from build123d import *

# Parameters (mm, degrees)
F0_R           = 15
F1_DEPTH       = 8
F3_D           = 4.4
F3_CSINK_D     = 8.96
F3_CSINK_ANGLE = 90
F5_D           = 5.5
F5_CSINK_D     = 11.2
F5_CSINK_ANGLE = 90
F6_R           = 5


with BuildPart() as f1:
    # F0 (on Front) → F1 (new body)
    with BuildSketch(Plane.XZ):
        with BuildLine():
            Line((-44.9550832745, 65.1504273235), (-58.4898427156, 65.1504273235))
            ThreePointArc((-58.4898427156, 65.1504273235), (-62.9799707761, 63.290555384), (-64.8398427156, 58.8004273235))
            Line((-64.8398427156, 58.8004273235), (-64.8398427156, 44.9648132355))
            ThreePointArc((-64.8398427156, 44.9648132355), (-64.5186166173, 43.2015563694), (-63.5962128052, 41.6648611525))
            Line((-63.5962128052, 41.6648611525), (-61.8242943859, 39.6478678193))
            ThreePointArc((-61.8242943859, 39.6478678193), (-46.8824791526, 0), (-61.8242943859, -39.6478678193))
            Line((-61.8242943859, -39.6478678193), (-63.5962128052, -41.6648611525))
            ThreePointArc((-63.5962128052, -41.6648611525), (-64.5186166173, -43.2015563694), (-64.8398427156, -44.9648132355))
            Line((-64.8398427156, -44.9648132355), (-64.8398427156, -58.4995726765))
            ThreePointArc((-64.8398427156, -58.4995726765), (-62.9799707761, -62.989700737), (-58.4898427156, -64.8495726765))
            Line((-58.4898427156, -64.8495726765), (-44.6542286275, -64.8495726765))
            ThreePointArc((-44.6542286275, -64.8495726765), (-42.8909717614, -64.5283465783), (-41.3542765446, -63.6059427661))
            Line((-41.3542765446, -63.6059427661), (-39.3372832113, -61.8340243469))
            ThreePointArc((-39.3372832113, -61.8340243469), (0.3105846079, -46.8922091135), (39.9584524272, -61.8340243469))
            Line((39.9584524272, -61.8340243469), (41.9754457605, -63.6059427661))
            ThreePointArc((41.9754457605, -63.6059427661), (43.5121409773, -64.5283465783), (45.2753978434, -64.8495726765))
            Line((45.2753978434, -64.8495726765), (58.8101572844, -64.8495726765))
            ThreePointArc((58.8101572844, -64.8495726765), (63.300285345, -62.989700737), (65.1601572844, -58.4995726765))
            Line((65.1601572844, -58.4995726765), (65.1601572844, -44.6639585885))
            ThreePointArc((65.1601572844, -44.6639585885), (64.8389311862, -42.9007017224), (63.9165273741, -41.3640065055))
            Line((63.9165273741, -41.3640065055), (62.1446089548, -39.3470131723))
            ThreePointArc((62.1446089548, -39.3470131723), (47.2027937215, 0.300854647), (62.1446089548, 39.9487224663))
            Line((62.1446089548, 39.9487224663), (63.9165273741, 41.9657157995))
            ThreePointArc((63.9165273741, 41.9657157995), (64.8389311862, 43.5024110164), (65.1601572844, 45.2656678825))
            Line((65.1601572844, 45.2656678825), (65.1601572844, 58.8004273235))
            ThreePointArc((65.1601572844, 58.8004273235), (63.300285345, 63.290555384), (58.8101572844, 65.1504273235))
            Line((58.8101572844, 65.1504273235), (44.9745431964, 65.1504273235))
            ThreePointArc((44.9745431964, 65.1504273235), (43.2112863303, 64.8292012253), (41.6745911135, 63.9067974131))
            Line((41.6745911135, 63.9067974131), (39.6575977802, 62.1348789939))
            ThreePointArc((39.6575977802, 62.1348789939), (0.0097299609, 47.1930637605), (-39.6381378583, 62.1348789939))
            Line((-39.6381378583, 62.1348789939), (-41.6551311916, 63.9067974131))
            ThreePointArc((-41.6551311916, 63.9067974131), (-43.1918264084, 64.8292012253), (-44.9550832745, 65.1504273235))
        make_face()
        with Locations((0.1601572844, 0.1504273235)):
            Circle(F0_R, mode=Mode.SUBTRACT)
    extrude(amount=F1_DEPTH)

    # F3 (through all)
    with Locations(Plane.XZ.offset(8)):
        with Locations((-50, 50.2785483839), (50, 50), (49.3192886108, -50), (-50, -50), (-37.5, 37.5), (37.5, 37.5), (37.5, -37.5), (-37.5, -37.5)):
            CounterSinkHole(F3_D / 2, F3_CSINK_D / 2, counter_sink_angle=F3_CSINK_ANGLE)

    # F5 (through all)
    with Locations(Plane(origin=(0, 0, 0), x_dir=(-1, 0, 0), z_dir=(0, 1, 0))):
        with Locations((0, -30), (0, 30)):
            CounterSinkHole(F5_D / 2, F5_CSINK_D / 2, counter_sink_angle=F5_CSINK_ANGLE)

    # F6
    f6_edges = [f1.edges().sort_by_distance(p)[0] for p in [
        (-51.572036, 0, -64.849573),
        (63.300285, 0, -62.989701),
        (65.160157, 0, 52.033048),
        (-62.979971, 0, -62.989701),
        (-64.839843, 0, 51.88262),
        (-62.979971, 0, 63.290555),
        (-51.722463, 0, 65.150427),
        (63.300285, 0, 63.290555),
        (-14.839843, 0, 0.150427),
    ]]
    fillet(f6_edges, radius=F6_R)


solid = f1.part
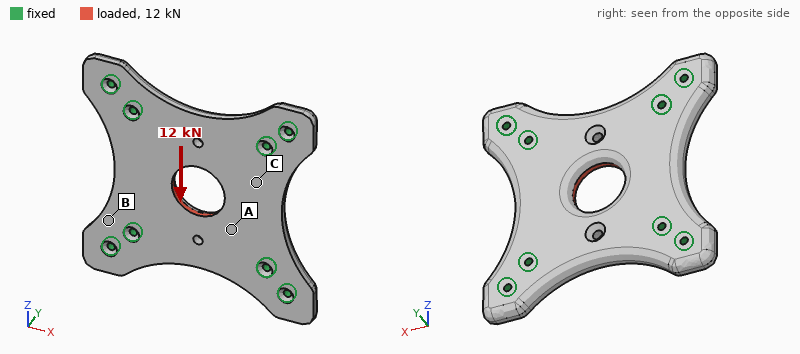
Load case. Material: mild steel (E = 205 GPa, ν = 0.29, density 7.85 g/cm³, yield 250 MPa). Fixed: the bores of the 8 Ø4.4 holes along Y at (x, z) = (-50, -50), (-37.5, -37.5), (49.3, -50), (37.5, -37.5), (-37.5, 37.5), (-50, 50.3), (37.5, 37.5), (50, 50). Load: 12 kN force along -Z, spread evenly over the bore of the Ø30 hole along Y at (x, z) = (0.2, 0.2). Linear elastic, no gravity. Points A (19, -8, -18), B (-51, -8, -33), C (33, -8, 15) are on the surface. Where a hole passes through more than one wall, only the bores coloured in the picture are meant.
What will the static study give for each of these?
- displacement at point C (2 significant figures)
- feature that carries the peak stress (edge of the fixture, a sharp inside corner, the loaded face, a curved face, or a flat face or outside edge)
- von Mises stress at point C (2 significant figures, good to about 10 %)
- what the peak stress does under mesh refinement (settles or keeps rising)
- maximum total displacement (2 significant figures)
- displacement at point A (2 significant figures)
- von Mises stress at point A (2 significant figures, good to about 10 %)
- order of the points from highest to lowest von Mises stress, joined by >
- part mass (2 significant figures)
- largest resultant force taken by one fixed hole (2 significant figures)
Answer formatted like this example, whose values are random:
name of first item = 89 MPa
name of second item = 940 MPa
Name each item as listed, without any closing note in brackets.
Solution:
displacement at point C = 1.7 µm
feature that carries the peak stress = edge of the fixture
von Mises stress at point C = 14 MPa
what the peak stress does under mesh refinement = keeps rising
maximum total displacement = 6.4 µm
displacement at point A = 3.3 µm
von Mises stress at point A = 23 MPa
order of the points from highest to lowest von Mises stress, joined by > = A > C > B
part mass = 710 g
largest resultant force taken by one fixed hole = 2.6 kN
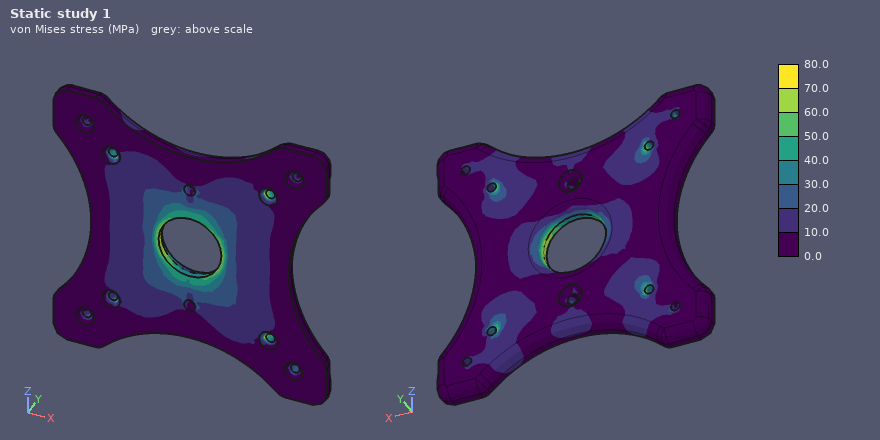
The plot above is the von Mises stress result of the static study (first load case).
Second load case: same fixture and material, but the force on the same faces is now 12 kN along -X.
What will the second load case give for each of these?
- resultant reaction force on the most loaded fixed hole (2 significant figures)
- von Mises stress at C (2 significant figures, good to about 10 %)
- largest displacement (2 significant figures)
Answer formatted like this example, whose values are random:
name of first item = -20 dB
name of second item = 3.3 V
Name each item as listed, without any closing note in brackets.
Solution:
resultant reaction force on the most loaded fixed hole = 2.6 kN
von Mises stress at C = 16 MPa
largest displacement = 6.4 µm
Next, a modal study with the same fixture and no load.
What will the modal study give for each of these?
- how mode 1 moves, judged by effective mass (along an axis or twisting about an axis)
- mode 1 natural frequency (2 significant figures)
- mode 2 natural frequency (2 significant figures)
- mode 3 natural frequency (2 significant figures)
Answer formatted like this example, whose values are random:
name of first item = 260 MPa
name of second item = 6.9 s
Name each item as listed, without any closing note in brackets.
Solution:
how mode 1 moves, judged by effective mass = along Y
mode 1 natural frequency = 4600 Hz
mode 2 natural frequency = 6900 Hz
mode 3 natural frequency = 6900 Hz
